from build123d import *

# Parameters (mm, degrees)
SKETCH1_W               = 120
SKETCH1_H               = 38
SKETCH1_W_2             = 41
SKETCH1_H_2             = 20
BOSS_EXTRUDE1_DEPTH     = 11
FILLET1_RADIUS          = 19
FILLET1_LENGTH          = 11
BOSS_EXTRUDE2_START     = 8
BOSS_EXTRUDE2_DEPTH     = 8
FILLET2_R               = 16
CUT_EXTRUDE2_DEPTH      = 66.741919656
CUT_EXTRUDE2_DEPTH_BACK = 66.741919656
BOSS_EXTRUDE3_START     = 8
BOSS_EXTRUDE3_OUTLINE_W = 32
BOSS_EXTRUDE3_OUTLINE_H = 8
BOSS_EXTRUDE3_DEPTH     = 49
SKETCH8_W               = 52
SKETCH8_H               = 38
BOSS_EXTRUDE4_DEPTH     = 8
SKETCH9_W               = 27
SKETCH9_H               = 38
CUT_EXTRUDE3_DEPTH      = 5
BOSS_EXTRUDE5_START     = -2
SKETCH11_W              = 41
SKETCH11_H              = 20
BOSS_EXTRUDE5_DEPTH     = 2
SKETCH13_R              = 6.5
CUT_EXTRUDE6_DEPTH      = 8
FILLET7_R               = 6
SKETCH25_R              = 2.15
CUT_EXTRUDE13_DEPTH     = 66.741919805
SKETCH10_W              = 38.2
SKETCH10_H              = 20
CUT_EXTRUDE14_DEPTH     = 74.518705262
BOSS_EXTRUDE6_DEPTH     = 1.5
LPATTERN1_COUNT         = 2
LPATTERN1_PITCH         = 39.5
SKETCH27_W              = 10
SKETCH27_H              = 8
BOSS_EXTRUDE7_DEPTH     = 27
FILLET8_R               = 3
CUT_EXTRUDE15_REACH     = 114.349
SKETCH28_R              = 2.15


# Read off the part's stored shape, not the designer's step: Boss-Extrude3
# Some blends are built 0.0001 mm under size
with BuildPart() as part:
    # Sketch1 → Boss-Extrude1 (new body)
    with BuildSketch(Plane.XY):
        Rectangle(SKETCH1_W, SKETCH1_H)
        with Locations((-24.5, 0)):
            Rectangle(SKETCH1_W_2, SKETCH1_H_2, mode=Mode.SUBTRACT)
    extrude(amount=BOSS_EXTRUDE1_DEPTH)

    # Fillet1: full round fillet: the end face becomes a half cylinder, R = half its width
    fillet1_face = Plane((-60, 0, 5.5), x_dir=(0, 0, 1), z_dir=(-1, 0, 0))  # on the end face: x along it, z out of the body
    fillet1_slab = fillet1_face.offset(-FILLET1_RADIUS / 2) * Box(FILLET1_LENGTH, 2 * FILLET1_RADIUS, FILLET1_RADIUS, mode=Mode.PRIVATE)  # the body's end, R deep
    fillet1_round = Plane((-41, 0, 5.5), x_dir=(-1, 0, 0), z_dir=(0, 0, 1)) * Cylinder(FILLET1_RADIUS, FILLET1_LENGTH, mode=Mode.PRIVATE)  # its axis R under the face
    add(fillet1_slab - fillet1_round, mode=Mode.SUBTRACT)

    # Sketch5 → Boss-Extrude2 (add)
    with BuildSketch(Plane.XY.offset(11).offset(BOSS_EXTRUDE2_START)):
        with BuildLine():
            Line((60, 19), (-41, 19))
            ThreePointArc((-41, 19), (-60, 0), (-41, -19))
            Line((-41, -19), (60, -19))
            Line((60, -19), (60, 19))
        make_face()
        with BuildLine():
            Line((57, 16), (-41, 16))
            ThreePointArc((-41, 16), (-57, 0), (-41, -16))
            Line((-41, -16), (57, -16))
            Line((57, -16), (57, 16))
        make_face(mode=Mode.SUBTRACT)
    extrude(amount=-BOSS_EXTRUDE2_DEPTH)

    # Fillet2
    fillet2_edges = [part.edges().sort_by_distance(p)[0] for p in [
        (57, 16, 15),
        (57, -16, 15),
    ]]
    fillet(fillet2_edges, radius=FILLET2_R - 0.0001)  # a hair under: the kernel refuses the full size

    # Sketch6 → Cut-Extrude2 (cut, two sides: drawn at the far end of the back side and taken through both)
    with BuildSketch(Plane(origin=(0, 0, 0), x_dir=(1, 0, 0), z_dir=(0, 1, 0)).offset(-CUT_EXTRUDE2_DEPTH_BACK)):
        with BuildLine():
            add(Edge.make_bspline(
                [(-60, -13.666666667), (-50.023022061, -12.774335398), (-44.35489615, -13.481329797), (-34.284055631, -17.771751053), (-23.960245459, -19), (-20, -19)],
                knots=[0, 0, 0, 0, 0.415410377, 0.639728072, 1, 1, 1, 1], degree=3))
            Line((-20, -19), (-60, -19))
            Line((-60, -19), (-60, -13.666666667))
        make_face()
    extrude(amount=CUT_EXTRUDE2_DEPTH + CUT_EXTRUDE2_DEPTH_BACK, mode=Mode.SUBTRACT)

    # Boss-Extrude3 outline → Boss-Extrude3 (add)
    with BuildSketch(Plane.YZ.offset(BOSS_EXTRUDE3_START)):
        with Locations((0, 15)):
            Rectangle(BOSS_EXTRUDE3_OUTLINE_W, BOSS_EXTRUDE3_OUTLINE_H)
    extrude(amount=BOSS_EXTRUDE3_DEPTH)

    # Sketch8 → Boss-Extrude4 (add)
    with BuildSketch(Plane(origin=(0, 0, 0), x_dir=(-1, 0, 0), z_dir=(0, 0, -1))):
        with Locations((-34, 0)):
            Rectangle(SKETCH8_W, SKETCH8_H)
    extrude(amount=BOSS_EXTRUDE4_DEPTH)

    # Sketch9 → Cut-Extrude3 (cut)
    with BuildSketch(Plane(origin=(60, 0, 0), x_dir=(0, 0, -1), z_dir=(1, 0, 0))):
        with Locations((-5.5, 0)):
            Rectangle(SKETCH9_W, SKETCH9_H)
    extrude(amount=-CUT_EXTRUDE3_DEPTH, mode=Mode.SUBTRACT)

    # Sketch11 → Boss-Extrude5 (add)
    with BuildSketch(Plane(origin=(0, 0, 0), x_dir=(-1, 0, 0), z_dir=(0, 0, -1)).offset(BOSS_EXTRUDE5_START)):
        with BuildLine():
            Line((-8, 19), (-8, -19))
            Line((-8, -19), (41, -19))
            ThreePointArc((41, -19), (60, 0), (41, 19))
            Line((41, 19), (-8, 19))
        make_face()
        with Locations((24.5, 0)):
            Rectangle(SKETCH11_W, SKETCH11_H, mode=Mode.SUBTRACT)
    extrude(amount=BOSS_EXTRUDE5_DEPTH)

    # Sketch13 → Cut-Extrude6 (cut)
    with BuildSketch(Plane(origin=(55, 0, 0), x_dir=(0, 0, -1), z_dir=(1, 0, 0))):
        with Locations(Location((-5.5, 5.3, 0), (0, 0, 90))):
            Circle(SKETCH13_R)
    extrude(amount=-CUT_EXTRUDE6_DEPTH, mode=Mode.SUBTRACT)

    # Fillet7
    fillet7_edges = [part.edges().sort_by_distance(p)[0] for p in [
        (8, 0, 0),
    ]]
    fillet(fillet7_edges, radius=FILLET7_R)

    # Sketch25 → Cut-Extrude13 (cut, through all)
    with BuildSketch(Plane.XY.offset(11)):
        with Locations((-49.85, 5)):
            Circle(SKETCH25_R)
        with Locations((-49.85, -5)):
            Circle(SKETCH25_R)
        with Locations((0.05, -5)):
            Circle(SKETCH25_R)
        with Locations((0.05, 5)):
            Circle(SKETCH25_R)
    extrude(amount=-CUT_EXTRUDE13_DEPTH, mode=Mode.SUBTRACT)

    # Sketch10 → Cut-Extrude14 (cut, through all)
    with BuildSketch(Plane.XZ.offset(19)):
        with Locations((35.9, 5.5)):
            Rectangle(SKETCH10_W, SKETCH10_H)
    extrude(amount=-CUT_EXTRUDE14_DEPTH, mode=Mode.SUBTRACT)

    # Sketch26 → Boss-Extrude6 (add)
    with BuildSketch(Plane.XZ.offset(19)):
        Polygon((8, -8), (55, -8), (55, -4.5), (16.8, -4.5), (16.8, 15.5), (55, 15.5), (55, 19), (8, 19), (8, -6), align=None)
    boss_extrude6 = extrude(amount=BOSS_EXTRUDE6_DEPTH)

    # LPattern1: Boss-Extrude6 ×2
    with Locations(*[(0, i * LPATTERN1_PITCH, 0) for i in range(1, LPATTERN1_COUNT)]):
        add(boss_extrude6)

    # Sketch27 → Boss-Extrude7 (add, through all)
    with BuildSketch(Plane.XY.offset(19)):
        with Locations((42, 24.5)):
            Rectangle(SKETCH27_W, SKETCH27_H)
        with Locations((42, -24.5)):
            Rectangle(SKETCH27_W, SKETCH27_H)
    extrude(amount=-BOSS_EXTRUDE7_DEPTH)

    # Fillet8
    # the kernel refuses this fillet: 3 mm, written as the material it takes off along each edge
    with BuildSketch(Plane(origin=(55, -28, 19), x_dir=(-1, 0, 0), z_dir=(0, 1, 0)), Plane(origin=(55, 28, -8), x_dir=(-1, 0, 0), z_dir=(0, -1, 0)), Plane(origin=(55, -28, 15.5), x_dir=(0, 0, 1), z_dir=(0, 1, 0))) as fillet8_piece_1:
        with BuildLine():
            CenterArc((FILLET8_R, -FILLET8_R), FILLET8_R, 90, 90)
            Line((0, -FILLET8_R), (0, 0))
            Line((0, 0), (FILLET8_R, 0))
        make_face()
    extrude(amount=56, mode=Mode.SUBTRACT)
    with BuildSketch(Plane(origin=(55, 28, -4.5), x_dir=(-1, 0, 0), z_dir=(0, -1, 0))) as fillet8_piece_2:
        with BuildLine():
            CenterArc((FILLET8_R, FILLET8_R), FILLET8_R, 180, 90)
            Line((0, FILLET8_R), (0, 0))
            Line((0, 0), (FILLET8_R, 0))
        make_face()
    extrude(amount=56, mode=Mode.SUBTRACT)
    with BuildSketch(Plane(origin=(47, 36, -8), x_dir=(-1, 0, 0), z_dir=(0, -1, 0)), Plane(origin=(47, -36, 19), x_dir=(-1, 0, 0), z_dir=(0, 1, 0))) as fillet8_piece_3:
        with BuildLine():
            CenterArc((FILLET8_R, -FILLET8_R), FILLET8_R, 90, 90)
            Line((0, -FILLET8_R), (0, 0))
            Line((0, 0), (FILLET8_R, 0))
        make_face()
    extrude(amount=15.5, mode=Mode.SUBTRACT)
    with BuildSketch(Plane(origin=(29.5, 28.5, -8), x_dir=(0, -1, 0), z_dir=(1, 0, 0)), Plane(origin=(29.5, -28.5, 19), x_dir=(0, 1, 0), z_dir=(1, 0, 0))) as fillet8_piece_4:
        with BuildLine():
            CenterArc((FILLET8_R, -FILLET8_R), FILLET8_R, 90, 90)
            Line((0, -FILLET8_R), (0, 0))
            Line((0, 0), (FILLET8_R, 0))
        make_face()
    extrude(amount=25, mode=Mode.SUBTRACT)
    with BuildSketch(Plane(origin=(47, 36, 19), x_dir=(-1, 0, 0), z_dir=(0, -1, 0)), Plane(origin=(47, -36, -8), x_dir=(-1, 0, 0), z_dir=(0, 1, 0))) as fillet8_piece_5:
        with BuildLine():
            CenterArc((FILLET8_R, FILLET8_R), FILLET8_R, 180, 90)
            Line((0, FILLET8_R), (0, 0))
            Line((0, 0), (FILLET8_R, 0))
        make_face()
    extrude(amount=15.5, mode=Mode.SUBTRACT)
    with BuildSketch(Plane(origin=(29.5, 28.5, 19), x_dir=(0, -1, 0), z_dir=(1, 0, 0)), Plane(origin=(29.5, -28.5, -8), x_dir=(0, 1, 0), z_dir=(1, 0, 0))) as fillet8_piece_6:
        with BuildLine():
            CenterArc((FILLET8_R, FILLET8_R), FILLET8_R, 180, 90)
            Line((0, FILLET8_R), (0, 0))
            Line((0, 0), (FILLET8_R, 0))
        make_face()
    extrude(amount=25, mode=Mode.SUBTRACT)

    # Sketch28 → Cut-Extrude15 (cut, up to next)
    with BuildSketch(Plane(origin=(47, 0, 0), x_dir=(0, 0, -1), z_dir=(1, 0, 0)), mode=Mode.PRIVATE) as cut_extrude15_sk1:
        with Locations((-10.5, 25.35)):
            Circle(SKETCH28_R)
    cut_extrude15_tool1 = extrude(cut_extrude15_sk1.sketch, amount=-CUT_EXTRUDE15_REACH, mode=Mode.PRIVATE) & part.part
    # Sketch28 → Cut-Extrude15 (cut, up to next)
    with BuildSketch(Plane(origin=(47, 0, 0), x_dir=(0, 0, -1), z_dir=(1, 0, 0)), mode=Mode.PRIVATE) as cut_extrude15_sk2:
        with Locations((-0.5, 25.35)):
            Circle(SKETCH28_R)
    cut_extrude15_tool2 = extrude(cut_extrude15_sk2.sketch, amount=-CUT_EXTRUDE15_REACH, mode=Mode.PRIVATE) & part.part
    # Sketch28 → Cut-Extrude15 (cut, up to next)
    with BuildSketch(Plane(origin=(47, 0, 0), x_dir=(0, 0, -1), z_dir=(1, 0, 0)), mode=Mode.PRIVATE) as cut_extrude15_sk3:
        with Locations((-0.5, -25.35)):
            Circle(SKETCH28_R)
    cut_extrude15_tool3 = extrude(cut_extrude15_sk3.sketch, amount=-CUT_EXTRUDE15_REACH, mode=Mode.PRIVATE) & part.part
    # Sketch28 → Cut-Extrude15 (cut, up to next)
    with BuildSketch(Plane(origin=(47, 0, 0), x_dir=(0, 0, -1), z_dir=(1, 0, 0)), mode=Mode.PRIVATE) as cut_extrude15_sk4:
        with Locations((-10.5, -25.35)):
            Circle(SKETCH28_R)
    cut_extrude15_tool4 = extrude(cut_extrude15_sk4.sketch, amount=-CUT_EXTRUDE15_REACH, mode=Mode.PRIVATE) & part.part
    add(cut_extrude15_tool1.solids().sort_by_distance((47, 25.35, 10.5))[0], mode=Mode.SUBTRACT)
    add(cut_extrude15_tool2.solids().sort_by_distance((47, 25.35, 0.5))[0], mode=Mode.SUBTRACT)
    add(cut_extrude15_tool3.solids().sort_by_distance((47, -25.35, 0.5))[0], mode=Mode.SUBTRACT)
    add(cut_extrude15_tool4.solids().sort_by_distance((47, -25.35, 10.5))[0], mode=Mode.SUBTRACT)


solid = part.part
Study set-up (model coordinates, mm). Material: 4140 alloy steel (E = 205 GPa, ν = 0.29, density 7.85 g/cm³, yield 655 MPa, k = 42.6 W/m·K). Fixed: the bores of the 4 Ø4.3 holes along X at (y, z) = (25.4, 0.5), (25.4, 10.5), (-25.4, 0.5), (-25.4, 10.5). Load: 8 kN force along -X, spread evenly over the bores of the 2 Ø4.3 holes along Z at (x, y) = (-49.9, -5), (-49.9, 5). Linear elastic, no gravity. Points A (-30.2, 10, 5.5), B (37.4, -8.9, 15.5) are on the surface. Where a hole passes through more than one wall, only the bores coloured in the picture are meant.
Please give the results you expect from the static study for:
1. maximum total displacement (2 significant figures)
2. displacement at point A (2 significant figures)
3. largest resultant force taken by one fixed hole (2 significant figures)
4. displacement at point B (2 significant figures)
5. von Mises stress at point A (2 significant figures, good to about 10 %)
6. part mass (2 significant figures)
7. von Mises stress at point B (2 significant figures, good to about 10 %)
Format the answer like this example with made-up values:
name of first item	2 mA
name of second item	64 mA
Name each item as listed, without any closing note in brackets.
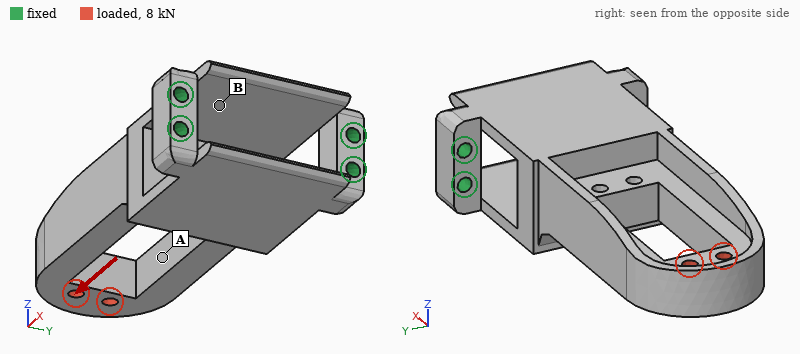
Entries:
maximum total displacement	43 µm
displacement at point A	24 µm
largest resultant force taken by one fixed hole	2.0 kN
displacement at point B	9.7 µm
von Mises stress at point A	65 MPa
part mass	350 g
von Mises stress at point B	21 MPa
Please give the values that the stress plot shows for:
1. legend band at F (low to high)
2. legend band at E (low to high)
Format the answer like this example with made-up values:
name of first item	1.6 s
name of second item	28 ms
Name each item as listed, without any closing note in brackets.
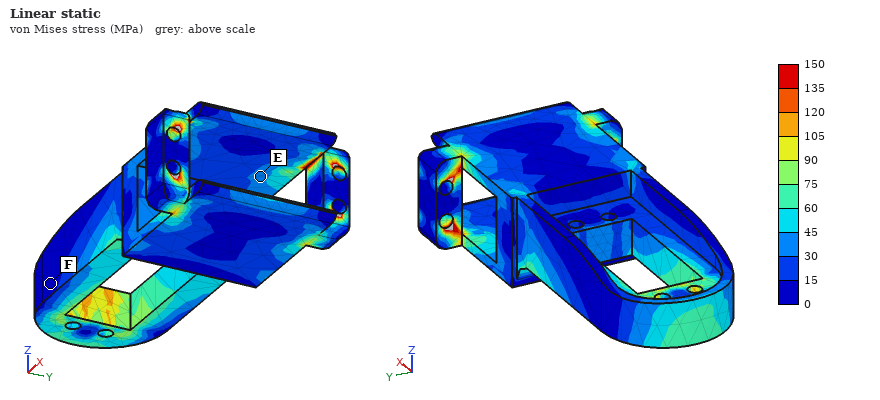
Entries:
legend band at F	0 to 15 MPa
legend band at E	30 to 45 MPa
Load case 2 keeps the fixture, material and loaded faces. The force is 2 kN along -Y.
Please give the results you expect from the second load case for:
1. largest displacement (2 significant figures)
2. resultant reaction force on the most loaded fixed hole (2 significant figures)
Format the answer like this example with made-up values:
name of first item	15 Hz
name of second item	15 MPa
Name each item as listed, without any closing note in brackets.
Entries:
largest displacement	0.19 mm
resultant reaction force on the most loaded fixed hole	2.2 kN
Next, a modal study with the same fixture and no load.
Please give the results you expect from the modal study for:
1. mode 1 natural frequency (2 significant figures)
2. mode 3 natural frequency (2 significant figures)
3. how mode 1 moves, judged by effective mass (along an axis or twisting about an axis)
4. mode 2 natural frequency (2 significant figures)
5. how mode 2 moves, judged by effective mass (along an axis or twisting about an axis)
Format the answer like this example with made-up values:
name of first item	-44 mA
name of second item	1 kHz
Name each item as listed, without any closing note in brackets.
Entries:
mode 1 natural frequency	1200 Hz
mode 3 natural frequency	3100 Hz
how mode 1 moves, judged by effective mass	along Z
mode 2 natural frequency	2000 Hz
how mode 2 moves, judged by effective mass	along Y
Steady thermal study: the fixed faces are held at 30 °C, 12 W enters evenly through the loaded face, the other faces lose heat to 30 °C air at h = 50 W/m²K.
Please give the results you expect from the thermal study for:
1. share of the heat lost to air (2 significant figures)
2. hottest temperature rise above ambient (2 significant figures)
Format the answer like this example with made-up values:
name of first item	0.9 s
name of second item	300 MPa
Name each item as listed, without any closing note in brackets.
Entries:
share of the heat lost to air	88 %
hottest temperature rise above ambient	47 K
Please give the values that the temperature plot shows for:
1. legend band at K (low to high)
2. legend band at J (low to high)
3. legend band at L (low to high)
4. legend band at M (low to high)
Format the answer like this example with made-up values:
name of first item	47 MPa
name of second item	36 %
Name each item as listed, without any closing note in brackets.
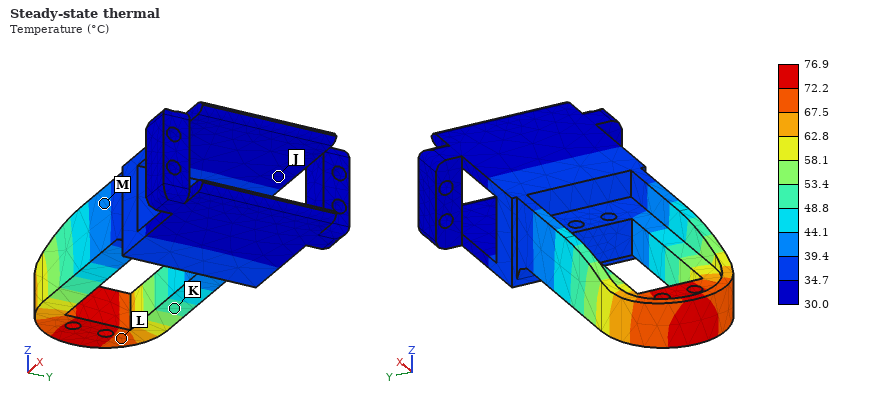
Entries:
legend band at K	48.8 to 53.4 °C
legend band at J	30.0 to 34.7 °C
legend band at L	67.5 to 72.2 °C
legend band at M	39.4 to 44.1 °C
